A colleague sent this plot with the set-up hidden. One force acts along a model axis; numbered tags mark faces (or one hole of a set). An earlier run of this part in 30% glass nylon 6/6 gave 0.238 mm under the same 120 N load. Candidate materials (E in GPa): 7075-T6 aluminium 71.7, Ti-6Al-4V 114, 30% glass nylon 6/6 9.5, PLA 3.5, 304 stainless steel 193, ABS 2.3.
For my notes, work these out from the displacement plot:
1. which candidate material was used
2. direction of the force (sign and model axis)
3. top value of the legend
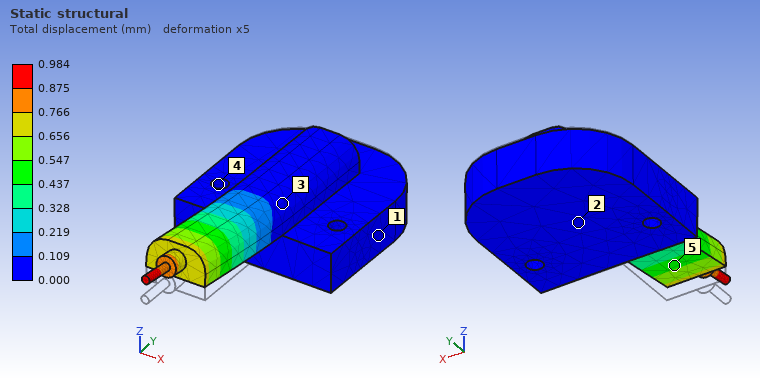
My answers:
ABS
+Z
0.984 mm
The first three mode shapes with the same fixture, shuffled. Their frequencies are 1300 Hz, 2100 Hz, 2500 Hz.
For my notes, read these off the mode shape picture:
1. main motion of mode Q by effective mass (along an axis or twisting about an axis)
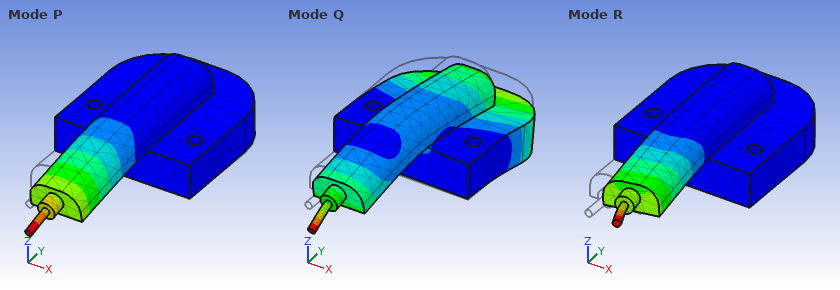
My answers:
along Z
